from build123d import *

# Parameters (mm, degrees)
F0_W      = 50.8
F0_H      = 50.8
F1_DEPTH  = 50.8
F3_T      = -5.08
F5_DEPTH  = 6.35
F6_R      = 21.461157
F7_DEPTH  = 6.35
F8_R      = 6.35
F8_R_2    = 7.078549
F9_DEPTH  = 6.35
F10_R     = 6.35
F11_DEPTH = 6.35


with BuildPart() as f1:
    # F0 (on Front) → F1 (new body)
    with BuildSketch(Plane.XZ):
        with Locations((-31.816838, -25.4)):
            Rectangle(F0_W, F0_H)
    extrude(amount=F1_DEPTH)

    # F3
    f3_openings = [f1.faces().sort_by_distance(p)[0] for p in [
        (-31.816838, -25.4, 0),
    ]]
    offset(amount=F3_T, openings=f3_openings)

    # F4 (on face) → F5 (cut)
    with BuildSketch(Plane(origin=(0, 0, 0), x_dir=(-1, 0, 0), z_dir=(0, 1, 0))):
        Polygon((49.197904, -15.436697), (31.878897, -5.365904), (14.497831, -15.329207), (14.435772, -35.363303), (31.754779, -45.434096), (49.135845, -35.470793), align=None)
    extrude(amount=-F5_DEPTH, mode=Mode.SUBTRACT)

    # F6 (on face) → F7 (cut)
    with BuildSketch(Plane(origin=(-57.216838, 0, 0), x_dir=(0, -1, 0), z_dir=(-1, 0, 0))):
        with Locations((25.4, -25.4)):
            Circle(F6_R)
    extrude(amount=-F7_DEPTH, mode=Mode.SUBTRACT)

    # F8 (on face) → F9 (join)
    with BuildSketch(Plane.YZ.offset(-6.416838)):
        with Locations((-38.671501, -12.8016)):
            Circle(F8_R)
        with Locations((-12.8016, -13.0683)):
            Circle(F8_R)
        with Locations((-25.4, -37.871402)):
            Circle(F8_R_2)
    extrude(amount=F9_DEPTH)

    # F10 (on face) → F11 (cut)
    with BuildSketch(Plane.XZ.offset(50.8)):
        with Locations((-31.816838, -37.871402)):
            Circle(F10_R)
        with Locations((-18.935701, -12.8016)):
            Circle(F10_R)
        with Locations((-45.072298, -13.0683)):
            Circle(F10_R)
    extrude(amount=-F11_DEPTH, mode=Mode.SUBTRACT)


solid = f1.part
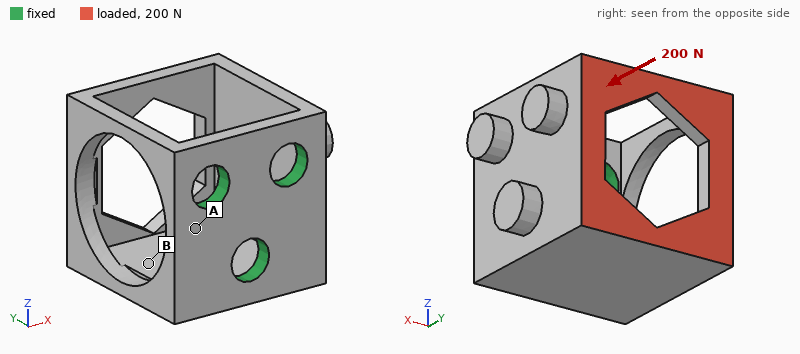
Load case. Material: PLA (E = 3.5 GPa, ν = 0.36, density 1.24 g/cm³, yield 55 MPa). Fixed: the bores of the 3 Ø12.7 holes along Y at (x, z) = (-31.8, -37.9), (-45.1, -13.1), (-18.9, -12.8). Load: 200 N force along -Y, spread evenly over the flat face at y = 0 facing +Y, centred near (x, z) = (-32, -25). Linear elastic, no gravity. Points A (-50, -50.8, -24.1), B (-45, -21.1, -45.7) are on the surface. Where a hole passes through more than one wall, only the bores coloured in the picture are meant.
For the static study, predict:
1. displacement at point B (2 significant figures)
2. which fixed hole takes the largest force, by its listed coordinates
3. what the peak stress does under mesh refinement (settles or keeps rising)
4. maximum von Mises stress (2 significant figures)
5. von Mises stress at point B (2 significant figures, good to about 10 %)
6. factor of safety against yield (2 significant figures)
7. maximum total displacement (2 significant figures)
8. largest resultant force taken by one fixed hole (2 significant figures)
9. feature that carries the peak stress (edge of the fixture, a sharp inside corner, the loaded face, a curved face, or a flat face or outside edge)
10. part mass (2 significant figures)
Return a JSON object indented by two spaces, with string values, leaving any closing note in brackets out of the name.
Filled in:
{
  "displacement at point B": "0.035 mm",
  "which fixed hole takes the largest force, by its listed coordinates": "(-31.8, -37.9)",
  "what the peak stress does under mesh refinement": "settles",
  "maximum von Mises stress": "9.3 MPa",
  "von Mises stress at point B": "1.7 MPa",
  "factor of safety against yield": "5.9",
  "maximum total displacement": "0.13 mm",
  "largest resultant force taken by one fixed hole": "95 N",
  "feature that carries the peak stress": "a curved face",
  "part mass": "54 g"
}
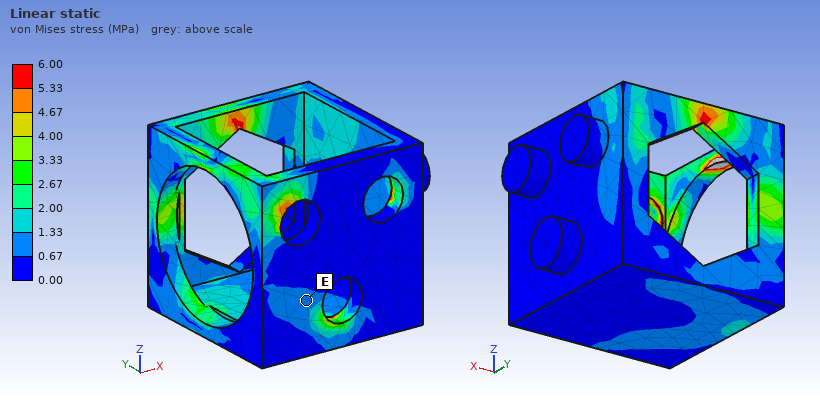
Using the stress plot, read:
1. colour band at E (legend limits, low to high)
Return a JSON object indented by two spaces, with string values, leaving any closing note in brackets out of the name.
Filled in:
{
  "colour band at E": "0.67 to 1.33 MPa"
}
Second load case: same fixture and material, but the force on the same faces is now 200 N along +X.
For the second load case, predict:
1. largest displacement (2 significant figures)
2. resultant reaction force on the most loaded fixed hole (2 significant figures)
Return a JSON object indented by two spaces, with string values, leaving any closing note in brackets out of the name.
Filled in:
{
  "largest displacement": "0.86 mm",
  "resultant reaction force on the most loaded fixed hole": "120 N"
}
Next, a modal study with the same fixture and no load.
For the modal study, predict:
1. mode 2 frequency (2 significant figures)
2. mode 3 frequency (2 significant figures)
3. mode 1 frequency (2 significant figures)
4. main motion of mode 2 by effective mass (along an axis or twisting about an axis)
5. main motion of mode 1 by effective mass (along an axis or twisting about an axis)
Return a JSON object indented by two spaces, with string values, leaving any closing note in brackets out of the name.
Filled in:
{
  "mode 2 frequency": "900 Hz",
  "mode 3 frequency": "2000 Hz",
  "mode 1 frequency": "640 Hz",
  "main motion of mode 2 by effective mass": "along Z",
  "main motion of mode 1 by effective mass": "along X"
}
